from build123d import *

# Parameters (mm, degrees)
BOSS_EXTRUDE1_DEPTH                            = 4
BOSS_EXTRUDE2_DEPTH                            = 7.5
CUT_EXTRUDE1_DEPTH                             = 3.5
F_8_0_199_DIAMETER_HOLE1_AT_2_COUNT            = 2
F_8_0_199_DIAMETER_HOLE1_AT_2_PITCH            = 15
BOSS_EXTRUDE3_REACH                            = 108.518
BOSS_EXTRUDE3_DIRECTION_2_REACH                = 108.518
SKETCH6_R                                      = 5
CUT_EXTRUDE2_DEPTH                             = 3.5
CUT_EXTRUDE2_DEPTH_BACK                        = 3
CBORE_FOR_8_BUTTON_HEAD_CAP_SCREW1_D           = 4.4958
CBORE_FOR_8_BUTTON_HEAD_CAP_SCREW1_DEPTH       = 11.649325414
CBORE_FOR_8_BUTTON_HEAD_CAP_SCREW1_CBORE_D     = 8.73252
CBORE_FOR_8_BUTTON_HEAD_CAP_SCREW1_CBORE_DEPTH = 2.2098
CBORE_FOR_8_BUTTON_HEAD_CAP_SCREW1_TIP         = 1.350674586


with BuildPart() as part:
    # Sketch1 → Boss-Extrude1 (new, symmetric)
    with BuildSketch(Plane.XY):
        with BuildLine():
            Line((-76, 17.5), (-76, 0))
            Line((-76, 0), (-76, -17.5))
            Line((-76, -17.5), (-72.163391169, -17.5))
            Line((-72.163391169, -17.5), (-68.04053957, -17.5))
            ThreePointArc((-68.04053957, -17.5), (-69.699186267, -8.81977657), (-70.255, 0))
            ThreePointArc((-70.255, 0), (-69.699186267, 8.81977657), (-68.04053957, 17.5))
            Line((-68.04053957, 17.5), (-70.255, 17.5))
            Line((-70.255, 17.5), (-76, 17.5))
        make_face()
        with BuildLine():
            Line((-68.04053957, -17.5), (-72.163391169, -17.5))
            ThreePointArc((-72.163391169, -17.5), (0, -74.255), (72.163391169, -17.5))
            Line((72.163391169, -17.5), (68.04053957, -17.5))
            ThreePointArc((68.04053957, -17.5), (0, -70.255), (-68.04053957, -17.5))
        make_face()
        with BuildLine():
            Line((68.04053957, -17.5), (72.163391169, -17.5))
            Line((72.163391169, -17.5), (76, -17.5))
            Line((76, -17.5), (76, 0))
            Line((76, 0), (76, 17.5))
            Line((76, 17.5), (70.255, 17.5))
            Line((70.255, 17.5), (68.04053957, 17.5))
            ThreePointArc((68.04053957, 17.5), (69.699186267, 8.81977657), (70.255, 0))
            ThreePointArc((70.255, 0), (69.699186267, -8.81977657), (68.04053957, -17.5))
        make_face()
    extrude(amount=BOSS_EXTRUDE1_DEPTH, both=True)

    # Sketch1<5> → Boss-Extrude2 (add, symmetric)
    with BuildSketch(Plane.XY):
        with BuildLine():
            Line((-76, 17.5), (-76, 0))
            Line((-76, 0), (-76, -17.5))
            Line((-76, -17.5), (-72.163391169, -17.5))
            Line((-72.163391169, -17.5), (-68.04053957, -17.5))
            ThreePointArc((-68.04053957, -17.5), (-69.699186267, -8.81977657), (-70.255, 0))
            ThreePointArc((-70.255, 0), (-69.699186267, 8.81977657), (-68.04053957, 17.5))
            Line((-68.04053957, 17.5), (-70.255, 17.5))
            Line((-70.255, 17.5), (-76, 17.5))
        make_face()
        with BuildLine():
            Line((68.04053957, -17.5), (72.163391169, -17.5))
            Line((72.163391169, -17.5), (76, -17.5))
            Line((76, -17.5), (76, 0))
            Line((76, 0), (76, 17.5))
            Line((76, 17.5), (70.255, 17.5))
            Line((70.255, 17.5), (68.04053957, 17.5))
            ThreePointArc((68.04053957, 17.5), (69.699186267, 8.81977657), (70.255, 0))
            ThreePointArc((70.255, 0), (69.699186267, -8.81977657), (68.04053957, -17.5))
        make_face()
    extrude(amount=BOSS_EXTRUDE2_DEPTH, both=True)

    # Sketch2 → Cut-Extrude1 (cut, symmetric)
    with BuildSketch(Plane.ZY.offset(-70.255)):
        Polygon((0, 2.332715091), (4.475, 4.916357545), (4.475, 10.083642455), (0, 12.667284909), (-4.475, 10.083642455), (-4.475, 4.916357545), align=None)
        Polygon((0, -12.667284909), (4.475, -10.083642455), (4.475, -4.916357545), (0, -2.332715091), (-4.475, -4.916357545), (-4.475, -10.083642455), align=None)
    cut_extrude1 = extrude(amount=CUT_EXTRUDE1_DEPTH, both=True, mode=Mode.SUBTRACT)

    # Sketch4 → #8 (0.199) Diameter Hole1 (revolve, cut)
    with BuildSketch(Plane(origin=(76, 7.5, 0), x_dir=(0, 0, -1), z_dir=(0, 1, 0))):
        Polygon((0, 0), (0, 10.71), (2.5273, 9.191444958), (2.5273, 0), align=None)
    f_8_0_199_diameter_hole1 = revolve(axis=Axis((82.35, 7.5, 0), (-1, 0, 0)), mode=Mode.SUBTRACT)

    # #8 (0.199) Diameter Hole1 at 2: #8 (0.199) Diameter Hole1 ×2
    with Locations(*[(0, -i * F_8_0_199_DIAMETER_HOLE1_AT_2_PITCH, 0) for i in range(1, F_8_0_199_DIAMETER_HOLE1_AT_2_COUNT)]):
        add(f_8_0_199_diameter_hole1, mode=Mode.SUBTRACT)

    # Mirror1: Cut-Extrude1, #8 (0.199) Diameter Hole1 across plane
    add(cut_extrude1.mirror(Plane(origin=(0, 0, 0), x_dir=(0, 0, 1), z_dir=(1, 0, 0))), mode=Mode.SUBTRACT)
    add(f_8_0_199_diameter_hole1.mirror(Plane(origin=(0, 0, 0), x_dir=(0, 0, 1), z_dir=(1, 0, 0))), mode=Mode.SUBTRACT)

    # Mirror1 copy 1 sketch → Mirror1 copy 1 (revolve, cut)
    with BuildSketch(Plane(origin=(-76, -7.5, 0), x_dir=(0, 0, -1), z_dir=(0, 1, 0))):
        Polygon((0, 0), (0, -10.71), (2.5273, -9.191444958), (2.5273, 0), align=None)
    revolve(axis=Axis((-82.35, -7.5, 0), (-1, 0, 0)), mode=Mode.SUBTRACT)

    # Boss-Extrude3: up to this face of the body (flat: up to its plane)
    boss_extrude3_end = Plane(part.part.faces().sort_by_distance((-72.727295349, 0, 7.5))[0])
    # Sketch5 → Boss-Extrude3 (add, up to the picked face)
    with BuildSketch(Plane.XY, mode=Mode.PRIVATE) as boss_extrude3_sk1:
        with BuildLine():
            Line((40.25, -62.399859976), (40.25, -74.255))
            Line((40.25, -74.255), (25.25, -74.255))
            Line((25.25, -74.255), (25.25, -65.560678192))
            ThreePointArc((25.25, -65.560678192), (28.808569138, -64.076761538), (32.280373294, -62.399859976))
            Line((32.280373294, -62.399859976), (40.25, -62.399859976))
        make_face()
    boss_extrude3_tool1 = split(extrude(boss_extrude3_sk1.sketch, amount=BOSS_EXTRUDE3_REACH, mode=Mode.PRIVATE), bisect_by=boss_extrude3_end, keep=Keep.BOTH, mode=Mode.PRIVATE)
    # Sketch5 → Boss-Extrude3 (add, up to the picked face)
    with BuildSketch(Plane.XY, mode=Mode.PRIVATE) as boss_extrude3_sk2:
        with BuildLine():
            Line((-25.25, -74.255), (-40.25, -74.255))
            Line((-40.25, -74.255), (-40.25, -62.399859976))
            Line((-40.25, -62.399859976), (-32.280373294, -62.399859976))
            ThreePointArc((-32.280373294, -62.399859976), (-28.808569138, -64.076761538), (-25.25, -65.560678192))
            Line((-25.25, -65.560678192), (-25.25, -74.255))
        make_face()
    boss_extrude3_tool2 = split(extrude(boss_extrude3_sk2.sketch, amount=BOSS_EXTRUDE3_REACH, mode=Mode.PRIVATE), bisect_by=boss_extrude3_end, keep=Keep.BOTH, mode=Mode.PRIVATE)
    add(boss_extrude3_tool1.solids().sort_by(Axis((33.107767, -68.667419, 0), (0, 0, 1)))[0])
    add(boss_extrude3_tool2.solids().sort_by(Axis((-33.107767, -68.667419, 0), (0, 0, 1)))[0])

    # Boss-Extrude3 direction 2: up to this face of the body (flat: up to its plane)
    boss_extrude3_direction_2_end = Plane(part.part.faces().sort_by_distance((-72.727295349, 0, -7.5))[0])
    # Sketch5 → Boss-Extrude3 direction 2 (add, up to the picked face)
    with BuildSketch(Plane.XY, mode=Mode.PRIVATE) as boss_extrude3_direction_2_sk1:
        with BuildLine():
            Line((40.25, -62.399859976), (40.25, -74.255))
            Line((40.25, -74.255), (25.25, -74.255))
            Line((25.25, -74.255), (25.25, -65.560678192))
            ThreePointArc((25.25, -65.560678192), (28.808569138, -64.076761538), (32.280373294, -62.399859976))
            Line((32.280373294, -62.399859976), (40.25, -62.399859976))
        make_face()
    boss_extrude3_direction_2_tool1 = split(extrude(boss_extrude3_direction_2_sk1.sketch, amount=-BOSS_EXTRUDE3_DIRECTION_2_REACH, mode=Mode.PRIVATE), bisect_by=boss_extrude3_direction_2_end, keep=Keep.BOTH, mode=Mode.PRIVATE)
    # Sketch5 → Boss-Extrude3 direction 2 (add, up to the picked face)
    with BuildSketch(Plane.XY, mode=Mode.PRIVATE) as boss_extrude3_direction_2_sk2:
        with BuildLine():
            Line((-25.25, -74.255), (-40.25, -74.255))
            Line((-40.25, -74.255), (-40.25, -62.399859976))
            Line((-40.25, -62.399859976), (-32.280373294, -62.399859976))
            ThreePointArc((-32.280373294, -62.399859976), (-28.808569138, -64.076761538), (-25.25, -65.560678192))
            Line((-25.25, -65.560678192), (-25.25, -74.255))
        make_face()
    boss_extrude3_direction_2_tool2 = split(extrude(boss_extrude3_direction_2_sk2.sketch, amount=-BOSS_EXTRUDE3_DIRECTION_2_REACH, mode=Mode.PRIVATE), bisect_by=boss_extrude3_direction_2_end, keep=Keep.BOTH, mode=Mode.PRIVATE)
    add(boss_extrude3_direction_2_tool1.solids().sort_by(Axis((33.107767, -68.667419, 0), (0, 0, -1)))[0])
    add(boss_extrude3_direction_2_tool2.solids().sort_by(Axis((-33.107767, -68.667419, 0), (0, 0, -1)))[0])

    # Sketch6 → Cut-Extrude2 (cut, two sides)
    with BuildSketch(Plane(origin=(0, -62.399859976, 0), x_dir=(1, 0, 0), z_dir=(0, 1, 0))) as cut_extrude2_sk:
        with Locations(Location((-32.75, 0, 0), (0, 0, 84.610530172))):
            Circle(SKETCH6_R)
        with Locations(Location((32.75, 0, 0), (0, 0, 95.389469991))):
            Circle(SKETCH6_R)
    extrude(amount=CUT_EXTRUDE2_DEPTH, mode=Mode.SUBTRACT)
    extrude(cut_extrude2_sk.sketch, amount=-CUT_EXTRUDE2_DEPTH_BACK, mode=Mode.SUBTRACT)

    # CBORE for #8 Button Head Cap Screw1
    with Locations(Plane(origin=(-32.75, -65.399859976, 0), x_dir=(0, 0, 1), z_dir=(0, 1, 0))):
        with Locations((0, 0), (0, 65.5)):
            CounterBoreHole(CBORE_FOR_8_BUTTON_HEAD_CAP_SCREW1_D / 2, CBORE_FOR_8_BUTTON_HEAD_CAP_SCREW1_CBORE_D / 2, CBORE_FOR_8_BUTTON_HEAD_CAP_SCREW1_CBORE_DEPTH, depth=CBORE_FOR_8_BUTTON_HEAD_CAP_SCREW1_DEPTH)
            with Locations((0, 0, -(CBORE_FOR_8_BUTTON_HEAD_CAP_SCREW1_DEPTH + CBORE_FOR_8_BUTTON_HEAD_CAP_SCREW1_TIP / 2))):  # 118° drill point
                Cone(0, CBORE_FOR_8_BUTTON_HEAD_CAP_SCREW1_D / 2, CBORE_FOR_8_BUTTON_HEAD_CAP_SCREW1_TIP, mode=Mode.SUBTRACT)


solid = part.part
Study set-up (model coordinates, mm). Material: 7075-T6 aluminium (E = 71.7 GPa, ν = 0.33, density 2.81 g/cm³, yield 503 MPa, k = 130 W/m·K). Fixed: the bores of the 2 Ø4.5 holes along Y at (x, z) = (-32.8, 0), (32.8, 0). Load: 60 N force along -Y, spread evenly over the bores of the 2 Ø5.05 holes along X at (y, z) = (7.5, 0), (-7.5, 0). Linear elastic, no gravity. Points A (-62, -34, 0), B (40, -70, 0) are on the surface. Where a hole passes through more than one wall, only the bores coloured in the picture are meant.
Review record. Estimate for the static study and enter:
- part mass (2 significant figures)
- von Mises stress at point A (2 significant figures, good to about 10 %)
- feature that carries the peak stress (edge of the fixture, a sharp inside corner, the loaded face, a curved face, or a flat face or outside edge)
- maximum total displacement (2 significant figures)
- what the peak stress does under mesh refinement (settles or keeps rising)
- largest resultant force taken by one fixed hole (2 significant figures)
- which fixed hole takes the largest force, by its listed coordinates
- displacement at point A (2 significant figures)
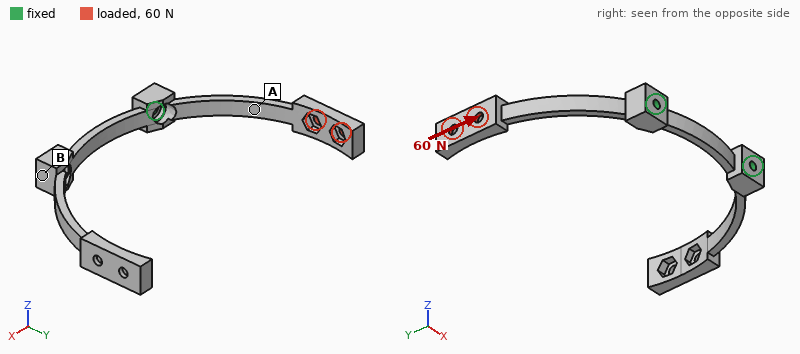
42 g
32 MPa
a sharp inside corner
1.7 mm
keeps rising
61 N
(-32.8, 0)
0.49 mm
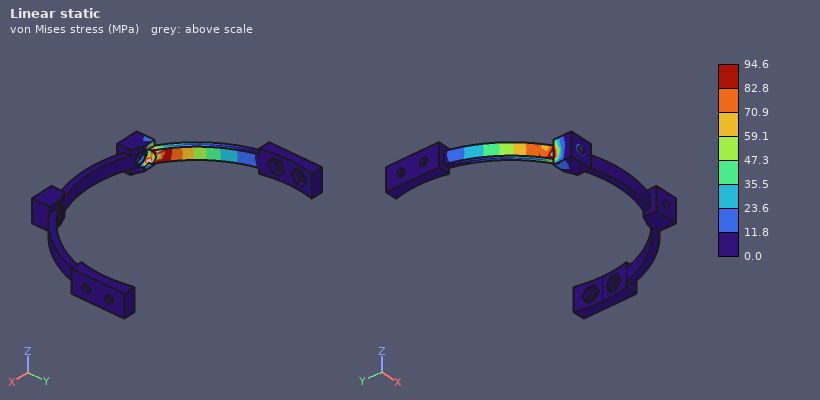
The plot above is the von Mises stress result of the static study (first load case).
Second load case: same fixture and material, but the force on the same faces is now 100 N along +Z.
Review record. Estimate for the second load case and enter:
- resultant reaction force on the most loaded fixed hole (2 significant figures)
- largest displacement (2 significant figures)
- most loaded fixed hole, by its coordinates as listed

110 N
2.1 mm
(-32.8, 0)
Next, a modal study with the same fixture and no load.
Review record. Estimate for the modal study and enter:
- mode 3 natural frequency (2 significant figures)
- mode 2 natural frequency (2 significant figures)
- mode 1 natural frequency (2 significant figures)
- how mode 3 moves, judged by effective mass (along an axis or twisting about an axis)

430 Hz
240 Hz
240 Hz
along Z
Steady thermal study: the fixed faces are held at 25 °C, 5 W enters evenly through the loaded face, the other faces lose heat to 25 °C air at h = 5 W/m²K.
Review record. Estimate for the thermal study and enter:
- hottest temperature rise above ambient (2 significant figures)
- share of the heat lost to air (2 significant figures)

74 K
18 %
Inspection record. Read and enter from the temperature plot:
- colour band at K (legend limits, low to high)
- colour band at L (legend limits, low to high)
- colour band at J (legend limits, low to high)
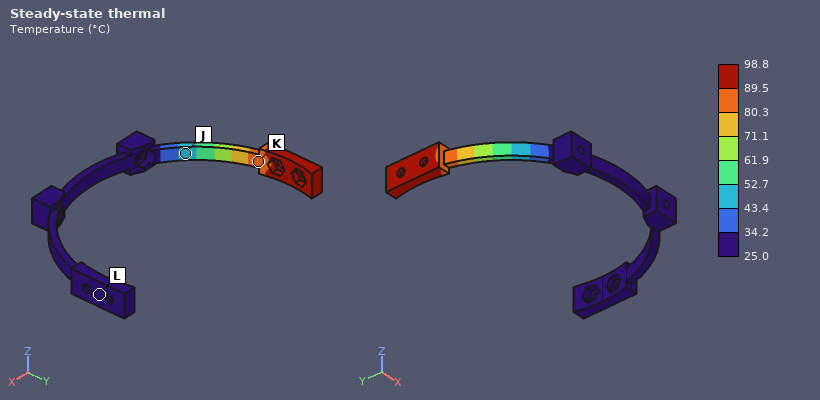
80.3 to 89.5 °C
25.0 to 34.2 °C
43.4 to 52.7 °C
